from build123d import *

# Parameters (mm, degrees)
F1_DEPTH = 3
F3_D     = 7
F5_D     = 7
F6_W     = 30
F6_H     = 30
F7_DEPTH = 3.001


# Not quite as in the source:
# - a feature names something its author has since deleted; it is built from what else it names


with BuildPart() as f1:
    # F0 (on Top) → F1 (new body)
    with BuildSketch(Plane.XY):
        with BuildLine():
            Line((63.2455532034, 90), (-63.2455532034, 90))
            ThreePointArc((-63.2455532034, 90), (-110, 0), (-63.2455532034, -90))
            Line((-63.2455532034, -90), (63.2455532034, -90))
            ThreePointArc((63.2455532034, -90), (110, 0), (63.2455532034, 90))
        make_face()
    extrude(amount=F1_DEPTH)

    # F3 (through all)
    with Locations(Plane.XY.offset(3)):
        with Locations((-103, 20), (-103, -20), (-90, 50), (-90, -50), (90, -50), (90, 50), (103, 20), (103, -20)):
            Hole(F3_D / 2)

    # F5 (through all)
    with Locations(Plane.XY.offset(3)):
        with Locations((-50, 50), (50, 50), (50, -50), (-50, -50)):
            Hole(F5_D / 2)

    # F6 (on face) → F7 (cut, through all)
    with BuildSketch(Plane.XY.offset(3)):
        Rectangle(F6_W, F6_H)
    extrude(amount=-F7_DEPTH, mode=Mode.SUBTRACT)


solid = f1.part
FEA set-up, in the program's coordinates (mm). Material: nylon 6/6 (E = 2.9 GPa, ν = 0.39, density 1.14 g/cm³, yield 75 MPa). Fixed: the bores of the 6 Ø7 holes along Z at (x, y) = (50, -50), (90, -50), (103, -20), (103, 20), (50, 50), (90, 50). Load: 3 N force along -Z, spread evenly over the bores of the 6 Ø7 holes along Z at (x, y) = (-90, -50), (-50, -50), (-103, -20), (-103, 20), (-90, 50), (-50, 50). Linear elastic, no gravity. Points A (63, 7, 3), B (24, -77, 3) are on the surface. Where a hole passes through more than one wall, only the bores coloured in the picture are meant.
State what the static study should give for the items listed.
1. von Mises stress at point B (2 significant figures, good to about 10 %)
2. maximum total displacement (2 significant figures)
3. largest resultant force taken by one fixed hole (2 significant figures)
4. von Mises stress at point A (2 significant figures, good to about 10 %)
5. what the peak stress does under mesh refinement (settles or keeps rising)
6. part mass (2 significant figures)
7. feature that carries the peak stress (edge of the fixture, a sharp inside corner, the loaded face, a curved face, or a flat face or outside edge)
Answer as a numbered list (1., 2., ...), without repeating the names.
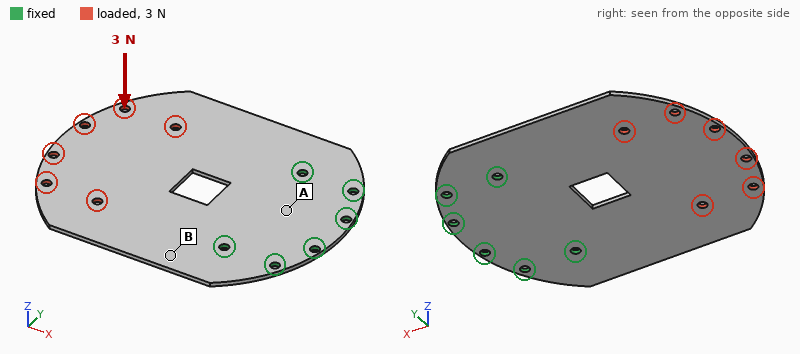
1. 1.2 MPa
2. 2.9 mm
3. 3.6 N
4. 0.42 MPa
5. keeps rising
6. 110 g
7. edge of the fixture
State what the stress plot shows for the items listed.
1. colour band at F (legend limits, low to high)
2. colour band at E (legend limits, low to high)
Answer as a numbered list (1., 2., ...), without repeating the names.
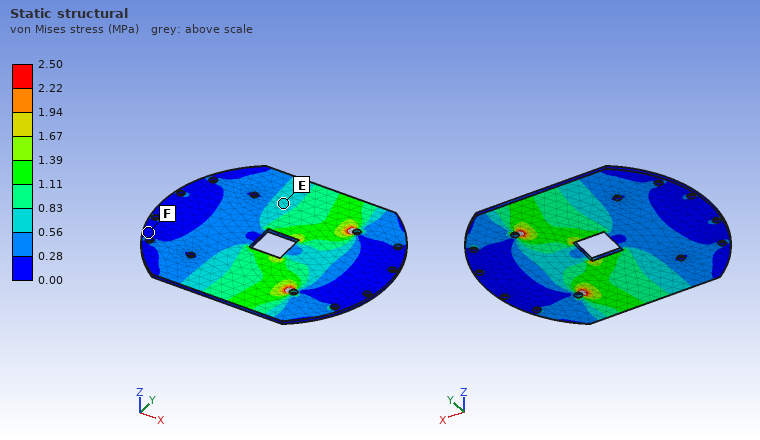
1. 0.00 to 0.28 MPa
2. 0.56 to 0.83 MPa
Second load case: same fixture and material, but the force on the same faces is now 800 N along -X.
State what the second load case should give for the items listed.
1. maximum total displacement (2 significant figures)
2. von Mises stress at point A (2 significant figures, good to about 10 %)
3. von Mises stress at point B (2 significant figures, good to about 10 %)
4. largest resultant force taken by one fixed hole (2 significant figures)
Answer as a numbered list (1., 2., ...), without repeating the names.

1. 0.13 mm
2. 0.65 MPa
3. 1.1 MPa
4. 270 N
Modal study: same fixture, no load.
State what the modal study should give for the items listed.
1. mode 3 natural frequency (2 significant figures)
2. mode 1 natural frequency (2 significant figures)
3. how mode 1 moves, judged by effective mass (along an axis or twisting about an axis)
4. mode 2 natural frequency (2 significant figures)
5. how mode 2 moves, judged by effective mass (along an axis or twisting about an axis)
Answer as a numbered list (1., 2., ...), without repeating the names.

1. 180 Hz
2. 34 Hz
3. along Z
4. 81 Hz
5. twisting about X
